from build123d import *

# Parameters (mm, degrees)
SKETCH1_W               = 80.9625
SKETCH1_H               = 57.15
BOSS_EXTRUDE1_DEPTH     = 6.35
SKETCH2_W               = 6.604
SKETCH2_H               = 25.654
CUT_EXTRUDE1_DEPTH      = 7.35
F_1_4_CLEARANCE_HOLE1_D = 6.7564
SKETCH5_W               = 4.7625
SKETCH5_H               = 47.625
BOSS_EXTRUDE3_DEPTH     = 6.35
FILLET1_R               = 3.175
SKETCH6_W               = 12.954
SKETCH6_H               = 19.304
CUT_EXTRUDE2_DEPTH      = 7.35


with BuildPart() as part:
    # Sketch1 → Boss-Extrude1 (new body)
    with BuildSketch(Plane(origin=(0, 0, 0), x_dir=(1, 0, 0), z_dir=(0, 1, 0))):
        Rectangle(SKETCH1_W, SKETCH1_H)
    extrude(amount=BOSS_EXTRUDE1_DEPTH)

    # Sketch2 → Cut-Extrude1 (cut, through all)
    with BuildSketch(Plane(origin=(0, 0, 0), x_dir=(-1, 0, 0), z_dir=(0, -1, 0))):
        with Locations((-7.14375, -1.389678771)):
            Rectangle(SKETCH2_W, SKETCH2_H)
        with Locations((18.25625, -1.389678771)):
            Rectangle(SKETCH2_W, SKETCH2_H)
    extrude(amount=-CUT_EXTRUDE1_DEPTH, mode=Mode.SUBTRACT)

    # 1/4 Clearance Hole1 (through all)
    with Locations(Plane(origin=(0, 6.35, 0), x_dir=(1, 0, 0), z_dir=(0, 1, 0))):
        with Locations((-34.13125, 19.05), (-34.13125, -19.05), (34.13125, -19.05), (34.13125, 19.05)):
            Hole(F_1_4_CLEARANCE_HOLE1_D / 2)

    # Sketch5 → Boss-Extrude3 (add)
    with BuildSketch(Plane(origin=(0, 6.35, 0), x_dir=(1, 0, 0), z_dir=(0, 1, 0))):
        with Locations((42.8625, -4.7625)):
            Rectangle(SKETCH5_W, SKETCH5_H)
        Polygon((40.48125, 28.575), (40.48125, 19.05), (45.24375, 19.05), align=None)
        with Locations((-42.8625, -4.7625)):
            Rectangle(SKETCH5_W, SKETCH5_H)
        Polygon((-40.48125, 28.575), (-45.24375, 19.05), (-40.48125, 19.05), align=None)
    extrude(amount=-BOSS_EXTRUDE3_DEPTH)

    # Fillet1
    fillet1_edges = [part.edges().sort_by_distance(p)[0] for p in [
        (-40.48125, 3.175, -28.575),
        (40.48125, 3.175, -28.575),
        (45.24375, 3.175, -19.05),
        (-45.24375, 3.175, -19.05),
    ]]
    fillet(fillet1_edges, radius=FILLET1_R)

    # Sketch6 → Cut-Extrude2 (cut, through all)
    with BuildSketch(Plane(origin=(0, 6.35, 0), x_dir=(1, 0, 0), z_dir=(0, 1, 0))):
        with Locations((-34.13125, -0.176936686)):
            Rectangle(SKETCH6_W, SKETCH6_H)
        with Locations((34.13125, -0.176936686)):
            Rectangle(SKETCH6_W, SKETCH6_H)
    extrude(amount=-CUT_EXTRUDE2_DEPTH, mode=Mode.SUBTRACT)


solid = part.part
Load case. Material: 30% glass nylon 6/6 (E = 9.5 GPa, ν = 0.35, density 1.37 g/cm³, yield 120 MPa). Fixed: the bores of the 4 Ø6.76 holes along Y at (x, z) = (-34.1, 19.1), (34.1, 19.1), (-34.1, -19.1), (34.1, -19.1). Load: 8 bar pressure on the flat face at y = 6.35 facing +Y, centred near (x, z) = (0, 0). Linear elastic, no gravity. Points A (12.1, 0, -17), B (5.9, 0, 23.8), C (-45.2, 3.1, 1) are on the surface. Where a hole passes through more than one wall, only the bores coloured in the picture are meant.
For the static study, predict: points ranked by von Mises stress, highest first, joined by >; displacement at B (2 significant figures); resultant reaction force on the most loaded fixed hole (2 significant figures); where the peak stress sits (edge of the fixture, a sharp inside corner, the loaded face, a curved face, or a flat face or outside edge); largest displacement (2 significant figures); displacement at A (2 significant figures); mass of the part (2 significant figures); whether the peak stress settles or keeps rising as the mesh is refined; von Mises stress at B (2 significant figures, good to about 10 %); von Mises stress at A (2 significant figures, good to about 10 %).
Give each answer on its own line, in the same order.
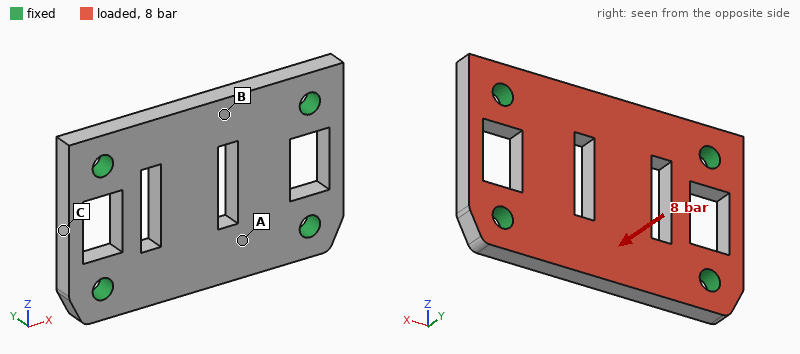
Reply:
B > A > C
0.25 mm
850 N
edge of the fixture
0.34 mm
0.21 mm
36 g
keeps rising
26 MPa
16 MPa
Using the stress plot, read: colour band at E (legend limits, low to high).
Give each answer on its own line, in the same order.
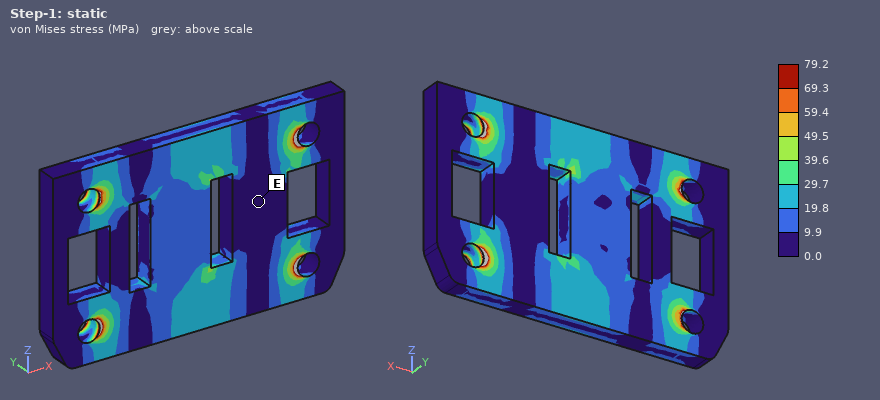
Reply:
0.0 to 9.9 MPa
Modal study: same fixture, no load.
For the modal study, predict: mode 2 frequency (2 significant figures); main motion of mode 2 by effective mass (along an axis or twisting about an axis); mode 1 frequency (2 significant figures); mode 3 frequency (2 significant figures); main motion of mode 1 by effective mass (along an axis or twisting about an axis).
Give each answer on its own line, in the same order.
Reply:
4400 Hz
twisting about X
3200 Hz
7000 Hz
along Y
